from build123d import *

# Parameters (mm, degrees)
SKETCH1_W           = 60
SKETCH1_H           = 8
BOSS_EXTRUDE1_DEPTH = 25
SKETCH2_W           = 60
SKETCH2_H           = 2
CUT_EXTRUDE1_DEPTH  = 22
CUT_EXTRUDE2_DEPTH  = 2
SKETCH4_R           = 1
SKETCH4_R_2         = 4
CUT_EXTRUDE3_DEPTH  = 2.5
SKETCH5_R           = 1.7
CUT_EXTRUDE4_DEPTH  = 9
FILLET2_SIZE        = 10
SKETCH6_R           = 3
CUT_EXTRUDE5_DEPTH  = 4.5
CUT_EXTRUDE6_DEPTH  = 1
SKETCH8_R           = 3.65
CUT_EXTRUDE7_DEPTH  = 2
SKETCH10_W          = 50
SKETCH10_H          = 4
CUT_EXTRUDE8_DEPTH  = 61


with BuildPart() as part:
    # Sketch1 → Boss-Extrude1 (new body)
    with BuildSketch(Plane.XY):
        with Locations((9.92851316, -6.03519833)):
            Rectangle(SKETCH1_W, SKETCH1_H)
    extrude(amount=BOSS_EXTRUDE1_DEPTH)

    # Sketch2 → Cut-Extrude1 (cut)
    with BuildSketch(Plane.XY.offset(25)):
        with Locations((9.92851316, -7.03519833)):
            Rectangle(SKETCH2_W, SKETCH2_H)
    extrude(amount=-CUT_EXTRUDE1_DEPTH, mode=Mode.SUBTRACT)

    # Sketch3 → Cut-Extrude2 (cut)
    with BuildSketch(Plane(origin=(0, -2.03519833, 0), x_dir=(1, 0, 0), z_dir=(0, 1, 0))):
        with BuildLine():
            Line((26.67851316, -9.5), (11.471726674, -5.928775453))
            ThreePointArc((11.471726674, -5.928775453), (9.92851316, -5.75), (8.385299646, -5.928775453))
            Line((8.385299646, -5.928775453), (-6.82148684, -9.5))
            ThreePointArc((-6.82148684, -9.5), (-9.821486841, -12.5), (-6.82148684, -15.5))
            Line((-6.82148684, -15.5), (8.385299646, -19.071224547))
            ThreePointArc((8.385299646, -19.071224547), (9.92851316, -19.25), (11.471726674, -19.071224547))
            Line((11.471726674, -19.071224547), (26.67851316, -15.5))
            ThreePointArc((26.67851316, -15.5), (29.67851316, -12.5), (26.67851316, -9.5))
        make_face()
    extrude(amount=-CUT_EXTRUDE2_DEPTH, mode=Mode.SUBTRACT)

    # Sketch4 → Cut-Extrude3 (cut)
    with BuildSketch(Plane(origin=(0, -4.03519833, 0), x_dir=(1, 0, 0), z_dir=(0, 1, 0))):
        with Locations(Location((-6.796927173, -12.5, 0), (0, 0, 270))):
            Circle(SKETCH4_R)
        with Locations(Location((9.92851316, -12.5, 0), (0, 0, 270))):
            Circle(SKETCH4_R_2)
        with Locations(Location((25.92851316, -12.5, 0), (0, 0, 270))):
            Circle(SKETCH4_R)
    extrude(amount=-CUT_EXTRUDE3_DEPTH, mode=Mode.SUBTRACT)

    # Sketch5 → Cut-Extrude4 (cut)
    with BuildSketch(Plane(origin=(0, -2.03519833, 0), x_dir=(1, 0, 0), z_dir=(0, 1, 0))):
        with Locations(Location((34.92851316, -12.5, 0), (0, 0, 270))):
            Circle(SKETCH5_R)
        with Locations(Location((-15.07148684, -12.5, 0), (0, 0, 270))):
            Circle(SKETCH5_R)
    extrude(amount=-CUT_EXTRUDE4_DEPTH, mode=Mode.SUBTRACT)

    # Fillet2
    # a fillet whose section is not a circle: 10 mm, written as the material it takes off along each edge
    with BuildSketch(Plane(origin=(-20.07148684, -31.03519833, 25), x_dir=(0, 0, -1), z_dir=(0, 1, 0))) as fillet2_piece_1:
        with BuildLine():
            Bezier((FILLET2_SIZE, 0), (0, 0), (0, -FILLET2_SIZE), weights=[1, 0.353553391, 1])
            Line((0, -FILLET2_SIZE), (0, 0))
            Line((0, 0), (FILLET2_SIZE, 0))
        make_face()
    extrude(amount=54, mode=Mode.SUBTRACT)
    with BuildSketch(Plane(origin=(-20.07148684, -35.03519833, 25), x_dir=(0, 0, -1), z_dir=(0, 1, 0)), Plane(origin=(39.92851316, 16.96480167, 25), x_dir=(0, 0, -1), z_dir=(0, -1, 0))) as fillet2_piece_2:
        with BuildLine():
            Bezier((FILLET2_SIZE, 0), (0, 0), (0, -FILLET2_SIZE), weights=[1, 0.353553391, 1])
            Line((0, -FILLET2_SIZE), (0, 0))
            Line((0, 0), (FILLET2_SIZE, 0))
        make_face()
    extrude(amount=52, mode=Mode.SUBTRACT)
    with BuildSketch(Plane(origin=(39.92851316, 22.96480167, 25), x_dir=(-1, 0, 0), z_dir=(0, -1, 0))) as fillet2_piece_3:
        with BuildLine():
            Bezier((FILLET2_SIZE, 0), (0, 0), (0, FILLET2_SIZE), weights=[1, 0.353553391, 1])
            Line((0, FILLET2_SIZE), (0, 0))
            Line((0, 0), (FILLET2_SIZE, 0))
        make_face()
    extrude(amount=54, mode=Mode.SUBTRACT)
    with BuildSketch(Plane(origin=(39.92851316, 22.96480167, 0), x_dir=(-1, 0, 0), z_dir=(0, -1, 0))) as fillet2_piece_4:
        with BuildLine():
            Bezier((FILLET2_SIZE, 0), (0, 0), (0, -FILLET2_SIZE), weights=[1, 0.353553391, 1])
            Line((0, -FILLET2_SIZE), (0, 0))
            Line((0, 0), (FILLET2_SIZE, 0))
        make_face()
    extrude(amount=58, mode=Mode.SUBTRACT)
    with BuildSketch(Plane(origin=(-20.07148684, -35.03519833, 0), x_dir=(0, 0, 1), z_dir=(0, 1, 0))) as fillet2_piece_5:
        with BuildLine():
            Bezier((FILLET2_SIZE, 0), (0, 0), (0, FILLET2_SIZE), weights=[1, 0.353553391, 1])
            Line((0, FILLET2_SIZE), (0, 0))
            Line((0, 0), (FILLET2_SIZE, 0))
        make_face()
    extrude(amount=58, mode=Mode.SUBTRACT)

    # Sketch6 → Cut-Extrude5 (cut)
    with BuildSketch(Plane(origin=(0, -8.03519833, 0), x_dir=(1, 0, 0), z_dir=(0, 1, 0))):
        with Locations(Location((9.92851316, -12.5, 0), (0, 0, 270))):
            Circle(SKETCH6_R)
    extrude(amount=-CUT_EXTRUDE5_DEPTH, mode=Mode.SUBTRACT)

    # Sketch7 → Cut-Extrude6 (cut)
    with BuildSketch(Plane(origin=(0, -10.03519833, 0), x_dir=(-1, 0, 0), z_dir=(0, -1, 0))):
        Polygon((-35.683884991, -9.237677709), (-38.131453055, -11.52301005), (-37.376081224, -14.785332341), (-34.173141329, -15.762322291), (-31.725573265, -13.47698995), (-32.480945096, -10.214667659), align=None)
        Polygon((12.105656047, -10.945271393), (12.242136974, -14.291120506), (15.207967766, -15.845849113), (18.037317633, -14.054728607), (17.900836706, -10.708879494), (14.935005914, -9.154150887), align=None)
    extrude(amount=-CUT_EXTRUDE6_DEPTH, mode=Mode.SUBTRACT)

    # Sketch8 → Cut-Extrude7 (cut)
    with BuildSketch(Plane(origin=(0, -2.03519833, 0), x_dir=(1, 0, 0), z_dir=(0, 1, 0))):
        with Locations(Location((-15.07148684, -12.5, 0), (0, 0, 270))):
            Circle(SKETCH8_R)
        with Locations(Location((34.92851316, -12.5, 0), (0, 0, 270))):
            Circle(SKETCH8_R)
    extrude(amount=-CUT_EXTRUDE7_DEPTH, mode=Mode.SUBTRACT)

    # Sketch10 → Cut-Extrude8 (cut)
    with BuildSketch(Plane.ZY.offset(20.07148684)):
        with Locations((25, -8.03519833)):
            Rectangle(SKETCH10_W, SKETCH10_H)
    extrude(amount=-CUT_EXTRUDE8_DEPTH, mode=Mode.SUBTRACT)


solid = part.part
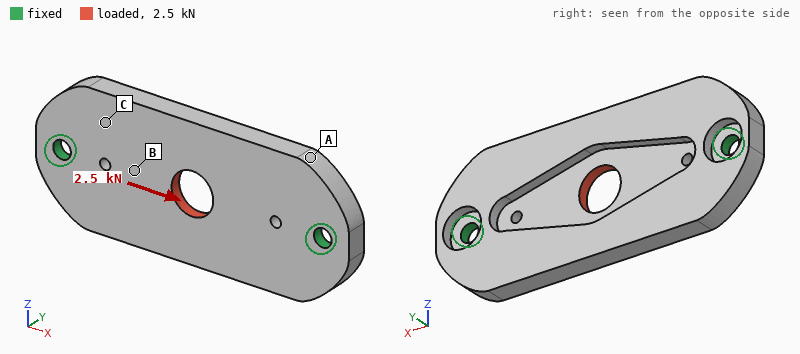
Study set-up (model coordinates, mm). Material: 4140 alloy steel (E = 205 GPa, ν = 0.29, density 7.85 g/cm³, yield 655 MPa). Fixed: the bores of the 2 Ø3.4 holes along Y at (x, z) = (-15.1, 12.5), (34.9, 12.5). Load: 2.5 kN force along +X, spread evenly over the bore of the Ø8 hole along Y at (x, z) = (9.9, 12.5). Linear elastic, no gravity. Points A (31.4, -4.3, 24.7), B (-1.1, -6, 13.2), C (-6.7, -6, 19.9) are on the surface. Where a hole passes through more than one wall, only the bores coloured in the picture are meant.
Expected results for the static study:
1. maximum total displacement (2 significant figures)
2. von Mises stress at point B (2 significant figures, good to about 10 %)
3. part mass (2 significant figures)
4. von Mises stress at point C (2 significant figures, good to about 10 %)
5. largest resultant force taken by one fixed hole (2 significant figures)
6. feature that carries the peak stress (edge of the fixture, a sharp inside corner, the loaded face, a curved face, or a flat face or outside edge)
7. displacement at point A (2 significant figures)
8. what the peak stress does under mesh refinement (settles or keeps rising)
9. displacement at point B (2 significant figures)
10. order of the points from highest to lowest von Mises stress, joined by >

4.8 µm
44 MPa
35 g
23 MPa
1.3 kN
edge of the fixture
2.7 µm
keeps rising
3.5 µm
B > C > A
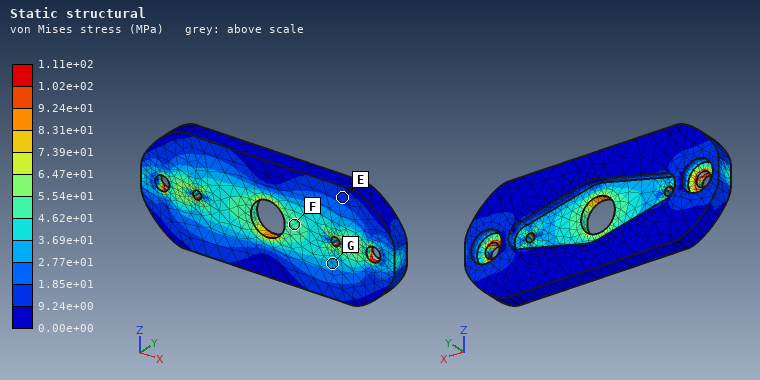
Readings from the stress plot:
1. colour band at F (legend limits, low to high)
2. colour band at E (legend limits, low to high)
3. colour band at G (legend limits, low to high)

4.62e+01 to 5.54e+01 MPa
9.24e+00 to 1.85e+01 MPa
2.77e+01 to 3.69e+01 MPa
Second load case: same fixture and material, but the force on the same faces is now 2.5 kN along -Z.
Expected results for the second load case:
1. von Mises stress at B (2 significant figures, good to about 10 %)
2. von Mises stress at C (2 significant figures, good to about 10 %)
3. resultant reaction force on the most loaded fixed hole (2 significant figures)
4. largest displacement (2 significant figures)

47 MPa
34 MPa
1.3 kN
14 µm
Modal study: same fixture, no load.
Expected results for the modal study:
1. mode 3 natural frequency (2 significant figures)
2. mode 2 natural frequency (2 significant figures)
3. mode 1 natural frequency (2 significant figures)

12 kHz
5600 Hz
5400 Hz
